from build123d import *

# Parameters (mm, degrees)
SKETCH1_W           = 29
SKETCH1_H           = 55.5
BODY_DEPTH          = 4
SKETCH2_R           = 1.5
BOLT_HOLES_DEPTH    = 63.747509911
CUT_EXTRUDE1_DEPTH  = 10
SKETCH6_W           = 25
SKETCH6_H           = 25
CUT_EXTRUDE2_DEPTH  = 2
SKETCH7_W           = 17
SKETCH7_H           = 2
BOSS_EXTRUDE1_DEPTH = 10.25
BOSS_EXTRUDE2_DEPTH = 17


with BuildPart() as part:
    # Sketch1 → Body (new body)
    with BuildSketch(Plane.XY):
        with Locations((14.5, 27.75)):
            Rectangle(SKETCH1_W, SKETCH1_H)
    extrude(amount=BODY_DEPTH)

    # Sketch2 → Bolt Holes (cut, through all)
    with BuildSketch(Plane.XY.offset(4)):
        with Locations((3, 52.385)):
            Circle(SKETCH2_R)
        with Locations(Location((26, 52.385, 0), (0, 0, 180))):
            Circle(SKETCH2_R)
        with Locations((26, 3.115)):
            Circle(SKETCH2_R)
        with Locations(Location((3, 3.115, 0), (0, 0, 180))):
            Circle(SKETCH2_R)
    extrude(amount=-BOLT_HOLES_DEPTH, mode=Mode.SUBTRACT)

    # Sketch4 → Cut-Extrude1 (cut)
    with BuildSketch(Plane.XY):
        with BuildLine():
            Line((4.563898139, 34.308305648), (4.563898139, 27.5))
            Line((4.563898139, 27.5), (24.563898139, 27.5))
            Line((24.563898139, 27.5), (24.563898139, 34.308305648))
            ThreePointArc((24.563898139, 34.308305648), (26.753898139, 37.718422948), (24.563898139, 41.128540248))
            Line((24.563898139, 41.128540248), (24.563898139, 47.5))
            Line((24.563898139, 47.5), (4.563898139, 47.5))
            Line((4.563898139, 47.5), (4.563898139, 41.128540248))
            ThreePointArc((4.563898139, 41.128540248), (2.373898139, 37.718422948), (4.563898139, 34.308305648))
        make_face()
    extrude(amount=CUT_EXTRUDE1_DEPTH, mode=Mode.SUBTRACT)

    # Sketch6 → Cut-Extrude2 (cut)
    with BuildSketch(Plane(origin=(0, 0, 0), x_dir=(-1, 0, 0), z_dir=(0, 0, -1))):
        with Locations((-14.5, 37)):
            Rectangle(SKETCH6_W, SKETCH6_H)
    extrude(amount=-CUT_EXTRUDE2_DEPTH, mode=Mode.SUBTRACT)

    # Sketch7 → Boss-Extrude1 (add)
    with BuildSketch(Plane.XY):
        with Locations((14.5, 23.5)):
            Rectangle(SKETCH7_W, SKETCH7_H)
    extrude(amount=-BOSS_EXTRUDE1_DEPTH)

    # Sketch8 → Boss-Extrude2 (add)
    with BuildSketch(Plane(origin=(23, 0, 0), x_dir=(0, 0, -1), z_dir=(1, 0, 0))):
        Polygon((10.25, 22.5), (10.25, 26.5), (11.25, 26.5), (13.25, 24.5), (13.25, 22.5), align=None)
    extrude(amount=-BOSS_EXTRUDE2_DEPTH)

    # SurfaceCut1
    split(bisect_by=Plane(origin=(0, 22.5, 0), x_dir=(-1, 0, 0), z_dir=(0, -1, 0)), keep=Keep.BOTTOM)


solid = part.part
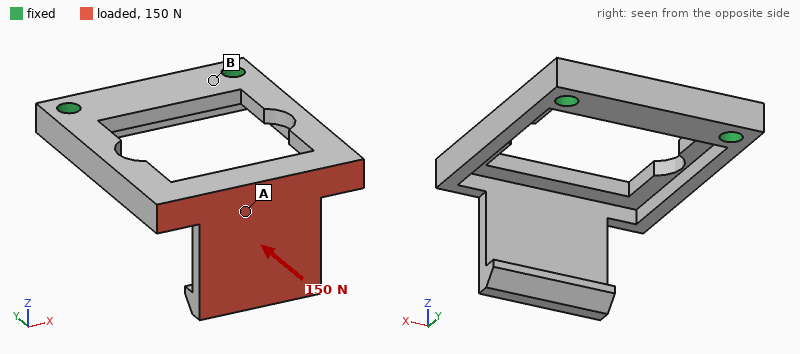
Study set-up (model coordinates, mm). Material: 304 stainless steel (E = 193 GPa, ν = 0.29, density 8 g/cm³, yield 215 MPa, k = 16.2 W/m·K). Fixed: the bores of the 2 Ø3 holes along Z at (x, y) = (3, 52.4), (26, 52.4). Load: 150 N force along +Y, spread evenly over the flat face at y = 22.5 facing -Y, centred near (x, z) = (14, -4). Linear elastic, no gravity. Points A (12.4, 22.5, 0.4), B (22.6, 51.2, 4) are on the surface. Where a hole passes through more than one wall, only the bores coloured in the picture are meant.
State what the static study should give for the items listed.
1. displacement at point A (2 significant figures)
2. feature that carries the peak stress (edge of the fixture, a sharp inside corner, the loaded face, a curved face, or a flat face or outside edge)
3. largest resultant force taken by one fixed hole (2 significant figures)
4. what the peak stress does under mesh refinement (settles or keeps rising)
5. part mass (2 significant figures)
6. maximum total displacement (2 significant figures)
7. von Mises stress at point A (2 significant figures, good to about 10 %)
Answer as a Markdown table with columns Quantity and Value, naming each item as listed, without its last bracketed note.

| Quantity | Value |
|---|---|
| displacement at point A | 0.074 mm |
| feature that carries the peak stress | a sharp inside corner |
| largest resultant force taken by one fixed hole | 75 N |
| what the peak stress does under mesh refinement | keeps rising |
| part mass | 18 g |
| maximum total displacement | 0.15 mm |
| von Mises stress at point A | 47 MPa |
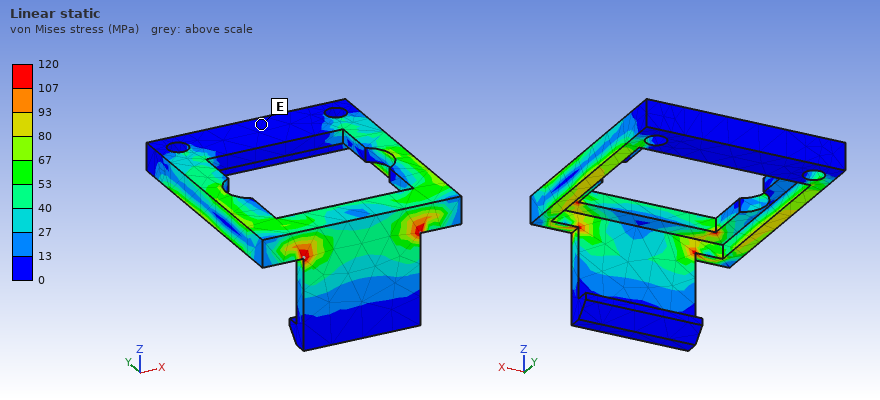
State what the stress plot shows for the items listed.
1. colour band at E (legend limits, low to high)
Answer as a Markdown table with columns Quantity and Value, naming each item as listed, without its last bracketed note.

| Quantity | Value |
|---|---|
| colour band at E | 0 to 13 MPa |
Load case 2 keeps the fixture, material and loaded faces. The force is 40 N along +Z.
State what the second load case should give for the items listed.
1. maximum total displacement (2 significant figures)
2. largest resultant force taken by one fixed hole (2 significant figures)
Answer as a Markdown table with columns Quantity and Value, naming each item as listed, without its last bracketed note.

| Quantity | Value |
|---|---|
| maximum total displacement | 77 µm |
| largest resultant force taken by one fixed hole | 20 N |
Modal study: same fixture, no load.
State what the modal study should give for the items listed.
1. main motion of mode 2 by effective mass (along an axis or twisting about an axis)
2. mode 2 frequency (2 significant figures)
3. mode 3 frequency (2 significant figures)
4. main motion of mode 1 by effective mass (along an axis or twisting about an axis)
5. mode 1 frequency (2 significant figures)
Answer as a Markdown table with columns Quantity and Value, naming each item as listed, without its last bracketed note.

| Quantity | Value |
|---|---|
| main motion of mode 2 by effective mass | along X |
| mode 2 frequency | 2200 Hz |
| mode 3 frequency | 3500 Hz |
| main motion of mode 1 by effective mass | along Z |
| mode 1 frequency | 1400 Hz |
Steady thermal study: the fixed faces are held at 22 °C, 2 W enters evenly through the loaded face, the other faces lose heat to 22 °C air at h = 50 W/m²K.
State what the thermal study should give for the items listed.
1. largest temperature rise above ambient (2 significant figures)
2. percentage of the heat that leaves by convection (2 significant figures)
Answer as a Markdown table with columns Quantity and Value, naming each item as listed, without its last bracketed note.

| Quantity | Value |
|---|---|
| largest temperature rise above ambient | 43 K |
| percentage of the heat that leaves by convection | 87 % |
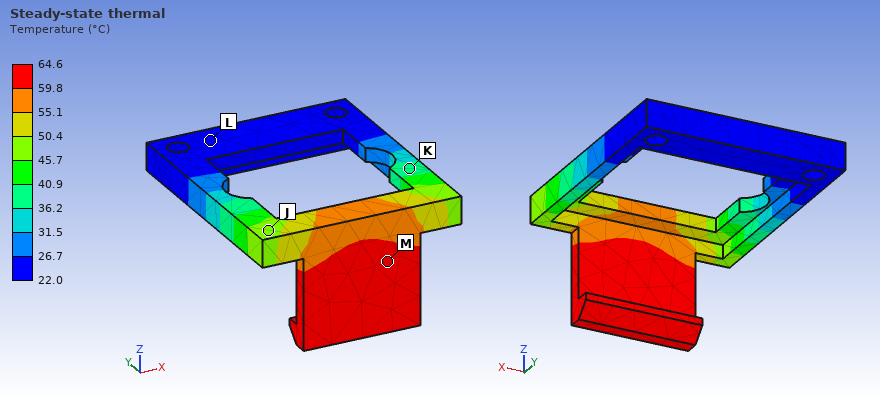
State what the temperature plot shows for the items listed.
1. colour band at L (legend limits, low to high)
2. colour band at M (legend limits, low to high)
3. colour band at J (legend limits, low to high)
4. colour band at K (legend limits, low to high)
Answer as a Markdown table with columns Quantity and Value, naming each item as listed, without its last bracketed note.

| Quantity | Value |
|---|---|
| colour band at L | 22.0 to 26.7 °C |
| colour band at M | 59.8 to 64.6 °C |
| colour band at J | 45.7 to 50.4 °C |
| colour band at K | 36.2 to 40.9 °C |
